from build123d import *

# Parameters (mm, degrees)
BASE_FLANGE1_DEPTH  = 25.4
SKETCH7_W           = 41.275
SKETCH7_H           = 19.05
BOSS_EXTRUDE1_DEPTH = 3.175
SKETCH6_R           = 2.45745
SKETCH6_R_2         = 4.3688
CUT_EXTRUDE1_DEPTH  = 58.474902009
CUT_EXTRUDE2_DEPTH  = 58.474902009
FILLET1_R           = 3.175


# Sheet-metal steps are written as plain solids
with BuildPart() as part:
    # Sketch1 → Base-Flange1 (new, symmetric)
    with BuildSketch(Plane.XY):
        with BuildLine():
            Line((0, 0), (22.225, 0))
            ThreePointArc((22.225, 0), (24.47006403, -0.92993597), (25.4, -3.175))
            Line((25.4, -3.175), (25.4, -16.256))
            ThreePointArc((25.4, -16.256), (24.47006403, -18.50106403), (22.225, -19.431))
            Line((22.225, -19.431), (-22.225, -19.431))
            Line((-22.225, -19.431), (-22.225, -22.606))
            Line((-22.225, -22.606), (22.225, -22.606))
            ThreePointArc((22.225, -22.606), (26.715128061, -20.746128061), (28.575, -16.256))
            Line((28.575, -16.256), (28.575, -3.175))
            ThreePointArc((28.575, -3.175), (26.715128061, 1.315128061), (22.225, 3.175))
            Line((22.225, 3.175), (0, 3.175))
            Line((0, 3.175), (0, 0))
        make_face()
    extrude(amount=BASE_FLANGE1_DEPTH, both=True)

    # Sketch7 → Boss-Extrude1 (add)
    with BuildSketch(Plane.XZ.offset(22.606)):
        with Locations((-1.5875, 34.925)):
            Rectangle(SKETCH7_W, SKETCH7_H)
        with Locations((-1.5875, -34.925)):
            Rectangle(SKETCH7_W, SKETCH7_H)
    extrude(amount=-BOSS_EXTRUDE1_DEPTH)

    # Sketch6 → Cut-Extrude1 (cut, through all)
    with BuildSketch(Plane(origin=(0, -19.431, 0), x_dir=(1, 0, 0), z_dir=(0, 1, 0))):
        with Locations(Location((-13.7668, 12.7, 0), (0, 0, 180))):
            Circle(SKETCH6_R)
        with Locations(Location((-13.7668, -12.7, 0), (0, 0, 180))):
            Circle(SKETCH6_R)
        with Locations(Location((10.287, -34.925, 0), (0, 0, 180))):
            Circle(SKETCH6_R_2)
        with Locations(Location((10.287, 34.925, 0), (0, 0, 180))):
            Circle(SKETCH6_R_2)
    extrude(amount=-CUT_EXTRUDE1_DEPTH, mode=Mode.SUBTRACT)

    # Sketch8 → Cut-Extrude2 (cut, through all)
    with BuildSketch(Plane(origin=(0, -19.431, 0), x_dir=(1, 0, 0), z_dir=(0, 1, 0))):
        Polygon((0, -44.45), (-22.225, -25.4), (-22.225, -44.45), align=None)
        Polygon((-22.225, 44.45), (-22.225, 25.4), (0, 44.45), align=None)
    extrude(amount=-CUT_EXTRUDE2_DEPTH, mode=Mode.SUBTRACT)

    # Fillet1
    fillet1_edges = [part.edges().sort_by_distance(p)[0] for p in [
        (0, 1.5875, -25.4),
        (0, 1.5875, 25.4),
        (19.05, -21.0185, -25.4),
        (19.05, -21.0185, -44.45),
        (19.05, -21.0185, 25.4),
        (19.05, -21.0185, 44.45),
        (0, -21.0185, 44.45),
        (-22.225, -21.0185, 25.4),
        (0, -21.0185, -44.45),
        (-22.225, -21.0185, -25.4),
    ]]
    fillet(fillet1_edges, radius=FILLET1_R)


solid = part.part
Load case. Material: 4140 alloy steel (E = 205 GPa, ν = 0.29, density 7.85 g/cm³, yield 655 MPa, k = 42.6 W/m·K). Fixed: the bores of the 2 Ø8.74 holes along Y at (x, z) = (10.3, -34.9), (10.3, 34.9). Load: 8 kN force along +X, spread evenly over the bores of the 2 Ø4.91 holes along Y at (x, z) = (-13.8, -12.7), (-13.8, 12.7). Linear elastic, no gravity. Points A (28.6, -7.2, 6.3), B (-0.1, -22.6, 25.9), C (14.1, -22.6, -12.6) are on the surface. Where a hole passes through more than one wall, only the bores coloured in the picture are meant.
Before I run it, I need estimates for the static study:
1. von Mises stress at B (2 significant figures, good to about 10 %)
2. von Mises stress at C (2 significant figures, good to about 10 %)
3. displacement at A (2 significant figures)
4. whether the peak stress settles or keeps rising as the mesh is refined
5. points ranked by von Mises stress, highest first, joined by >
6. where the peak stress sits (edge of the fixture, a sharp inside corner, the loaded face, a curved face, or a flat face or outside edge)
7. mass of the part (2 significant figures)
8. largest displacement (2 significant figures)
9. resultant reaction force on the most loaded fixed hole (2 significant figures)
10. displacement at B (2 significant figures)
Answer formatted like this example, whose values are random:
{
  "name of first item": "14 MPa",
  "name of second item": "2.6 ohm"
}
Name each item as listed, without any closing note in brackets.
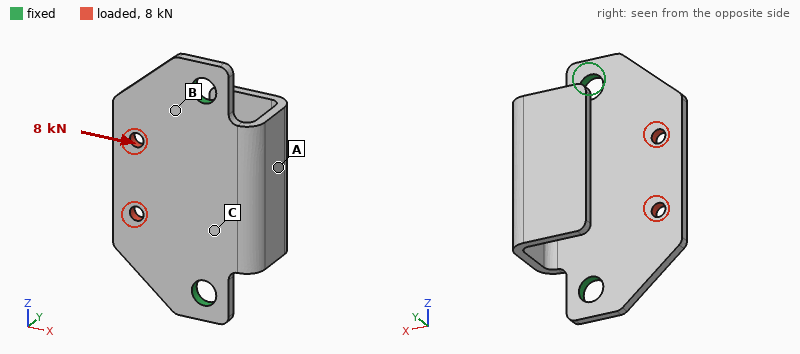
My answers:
{
  "von Mises stress at B": "71 MPa",
  "von Mises stress at C": "30 MPa",
  "displacement at A": "13 µm",
  "whether the peak stress settles or keeps rising as the mesh is refined": "keeps rising",
  "points ranked by von Mises stress, highest first, joined by >": "B > C > A",
  "where the peak stress sits": "edge of the fixture",
  "mass of the part": "140 g",
  "largest displacement": "17 µm",
  "resultant reaction force on the most loaded fixed hole": "4.2 kN",
  "displacement at B": "5.5 µm"
}
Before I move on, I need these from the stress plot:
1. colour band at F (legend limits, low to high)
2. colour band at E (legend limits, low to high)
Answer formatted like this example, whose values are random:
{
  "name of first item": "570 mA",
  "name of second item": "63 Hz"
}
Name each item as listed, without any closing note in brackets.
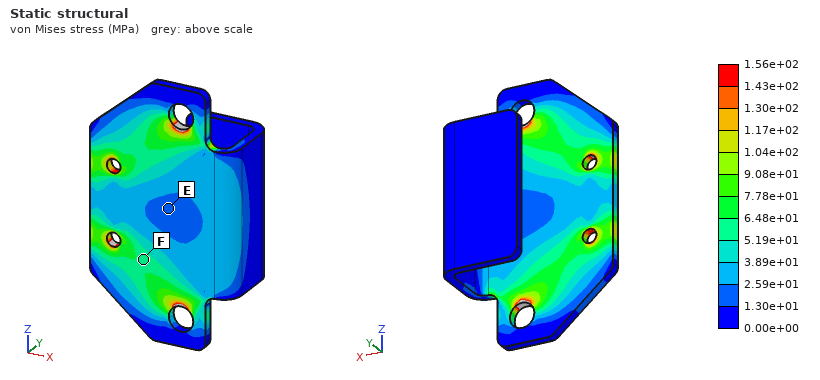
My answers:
{
  "colour band at F": "5.19e+01 to 6.48e+01 MPa",
  "colour band at E": "1.30e+01 to 2.59e+01 MPa"
}
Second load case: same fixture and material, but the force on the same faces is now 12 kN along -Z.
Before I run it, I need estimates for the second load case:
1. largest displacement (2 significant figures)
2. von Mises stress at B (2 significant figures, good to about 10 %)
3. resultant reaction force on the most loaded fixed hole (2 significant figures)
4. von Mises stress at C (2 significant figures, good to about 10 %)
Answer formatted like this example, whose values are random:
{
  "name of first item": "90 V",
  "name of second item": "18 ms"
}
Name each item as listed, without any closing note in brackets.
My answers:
{
  "largest displacement": "23 µm",
  "von Mises stress at B": "100 MPa",
  "resultant reaction force on the most loaded fixed hole": "7.1 kN",
  "von Mises stress at C": "30 MPa"
}
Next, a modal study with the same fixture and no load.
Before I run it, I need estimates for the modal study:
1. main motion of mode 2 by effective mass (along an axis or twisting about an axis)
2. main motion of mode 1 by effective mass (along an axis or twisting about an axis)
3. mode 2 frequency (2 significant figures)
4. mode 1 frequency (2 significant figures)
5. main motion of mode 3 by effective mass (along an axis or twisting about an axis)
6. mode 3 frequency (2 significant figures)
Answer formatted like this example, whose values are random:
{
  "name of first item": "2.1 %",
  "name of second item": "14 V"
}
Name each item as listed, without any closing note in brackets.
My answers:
{
  "main motion of mode 2 by effective mass": "along Z",
  "main motion of mode 1 by effective mass": "along X",
  "mode 2 frequency": "1800 Hz",
  "mode 1 frequency": "1000 Hz",
  "main motion of mode 3 by effective mass": "along Y",
  "mode 3 frequency": "2000 Hz"
}
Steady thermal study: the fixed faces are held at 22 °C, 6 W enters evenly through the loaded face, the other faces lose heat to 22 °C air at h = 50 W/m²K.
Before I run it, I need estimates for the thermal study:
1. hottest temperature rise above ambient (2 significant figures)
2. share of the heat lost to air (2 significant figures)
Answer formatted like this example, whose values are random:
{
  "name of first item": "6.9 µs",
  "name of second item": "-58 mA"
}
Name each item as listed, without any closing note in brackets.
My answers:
{
  "hottest temperature rise above ambient": "19 K",
  "share of the heat lost to air": "49 %"
}
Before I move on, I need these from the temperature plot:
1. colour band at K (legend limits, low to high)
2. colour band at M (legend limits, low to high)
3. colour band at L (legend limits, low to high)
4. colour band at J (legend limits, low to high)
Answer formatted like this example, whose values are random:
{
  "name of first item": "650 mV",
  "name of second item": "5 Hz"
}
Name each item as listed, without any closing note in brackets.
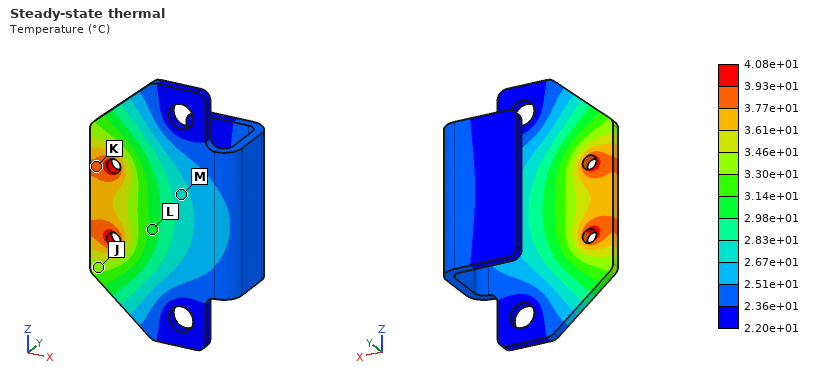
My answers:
{
  "colour band at K": "3.77e+01 to 3.93e+01 °C",
  "colour band at M": "2.67e+01 to 2.83e+01 °C",
  "colour band at L": "2.98e+01 to 3.14e+01 °C",
  "colour band at J": "3.30e+01 to 3.46e+01 °C"
}
